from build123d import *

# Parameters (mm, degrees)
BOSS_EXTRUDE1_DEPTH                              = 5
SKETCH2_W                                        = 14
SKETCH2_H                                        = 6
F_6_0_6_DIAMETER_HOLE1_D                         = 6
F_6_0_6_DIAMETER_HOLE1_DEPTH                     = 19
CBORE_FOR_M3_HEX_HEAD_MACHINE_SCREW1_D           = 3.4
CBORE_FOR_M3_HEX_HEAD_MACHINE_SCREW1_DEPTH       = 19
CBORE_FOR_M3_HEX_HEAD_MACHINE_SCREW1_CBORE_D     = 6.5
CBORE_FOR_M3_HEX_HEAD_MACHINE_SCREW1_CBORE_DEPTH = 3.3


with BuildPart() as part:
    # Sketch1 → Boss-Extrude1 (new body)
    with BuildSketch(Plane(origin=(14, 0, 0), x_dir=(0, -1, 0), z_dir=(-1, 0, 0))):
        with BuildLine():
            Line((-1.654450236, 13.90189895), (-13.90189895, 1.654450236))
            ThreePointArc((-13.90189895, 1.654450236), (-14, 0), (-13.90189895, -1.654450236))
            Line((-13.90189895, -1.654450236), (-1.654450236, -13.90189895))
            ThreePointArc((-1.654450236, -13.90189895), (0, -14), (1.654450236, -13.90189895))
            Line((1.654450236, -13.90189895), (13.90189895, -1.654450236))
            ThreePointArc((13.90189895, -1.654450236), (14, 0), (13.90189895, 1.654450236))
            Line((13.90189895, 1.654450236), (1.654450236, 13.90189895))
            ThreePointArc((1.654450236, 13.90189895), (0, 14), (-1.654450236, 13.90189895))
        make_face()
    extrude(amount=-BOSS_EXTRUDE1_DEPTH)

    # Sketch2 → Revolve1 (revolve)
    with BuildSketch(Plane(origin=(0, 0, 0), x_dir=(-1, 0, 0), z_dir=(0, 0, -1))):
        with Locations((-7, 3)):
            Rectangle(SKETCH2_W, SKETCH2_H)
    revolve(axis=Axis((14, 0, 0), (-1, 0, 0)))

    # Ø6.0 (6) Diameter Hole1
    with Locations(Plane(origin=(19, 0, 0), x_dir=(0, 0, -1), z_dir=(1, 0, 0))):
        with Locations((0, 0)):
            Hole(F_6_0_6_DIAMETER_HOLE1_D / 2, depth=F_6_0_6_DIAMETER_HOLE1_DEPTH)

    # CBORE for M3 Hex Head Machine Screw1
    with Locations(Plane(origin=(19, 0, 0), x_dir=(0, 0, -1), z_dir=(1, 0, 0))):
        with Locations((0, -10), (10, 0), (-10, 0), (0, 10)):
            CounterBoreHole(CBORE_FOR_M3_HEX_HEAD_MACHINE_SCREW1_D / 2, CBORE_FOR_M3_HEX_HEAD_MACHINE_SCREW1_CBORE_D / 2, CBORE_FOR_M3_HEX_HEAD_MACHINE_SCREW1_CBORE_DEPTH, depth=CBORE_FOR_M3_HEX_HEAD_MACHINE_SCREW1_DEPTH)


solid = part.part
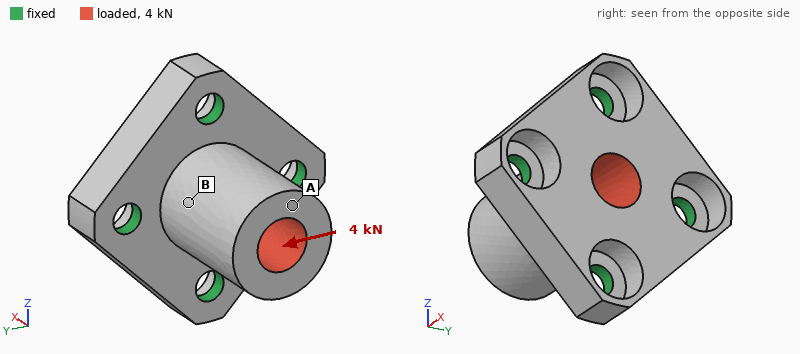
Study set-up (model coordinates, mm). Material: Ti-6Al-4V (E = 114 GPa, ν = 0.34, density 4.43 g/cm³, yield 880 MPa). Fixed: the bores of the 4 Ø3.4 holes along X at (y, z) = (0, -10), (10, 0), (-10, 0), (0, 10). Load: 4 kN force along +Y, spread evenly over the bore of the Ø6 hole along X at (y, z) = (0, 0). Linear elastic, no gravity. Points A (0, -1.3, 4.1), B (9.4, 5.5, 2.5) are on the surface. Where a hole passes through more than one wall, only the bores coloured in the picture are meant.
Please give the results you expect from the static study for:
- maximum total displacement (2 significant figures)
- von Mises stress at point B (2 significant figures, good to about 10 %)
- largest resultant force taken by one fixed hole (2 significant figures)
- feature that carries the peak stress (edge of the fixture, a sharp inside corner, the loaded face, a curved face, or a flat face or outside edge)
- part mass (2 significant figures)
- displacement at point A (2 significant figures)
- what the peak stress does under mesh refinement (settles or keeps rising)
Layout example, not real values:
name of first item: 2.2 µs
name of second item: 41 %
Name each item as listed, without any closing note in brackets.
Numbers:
maximum total displacement: 45 µm
von Mises stress at point B: 53 MPa
largest resultant force taken by one fixed hole: 1.6 kN
feature that carries the peak stress: edge of the fixture
part mass: 13 g
displacement at point A: 42 µm
what the peak stress does under mesh refinement: keeps rising
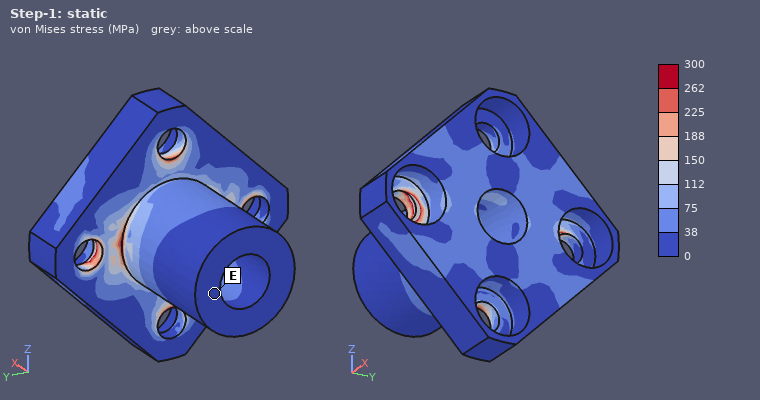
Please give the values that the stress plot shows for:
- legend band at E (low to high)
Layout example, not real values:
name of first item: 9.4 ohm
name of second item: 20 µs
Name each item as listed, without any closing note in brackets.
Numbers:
legend band at E: 0 to 38 MPa
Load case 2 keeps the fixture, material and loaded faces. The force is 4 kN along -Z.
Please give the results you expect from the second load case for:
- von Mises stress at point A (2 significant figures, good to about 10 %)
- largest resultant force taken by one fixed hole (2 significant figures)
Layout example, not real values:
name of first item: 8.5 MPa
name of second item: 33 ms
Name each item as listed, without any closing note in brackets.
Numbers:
von Mises stress at point A: 23 MPa
largest resultant force taken by one fixed hole: 1.6 kN
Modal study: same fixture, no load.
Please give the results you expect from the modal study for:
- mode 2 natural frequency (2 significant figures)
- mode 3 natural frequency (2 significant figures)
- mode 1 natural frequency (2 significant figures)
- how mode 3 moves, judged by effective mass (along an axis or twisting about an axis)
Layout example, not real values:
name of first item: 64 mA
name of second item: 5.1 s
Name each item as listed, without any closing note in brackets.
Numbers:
mode 2 natural frequency: 21 kHz
mode 3 natural frequency: 35 kHz
mode 1 natural frequency: 21 kHz
how mode 3 moves, judged by effective mass: along X
